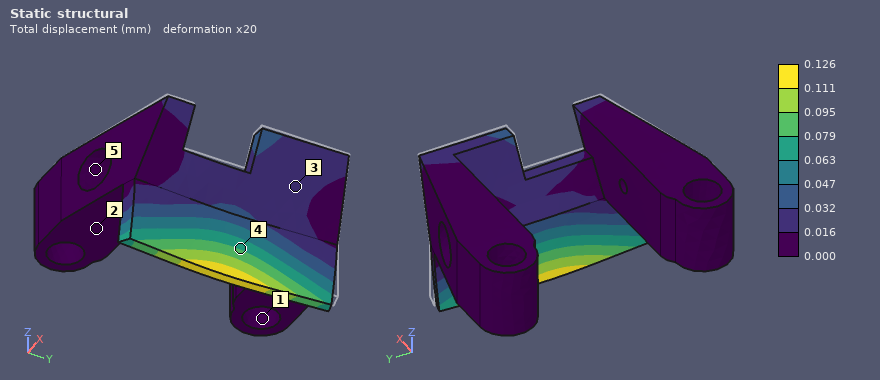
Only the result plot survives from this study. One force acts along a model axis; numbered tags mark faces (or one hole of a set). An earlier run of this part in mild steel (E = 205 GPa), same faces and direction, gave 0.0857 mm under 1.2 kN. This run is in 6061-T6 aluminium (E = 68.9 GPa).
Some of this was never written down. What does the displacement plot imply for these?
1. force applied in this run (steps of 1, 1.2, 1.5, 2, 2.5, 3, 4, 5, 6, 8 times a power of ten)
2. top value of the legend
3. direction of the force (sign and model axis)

600 N
0.126 mm
-X
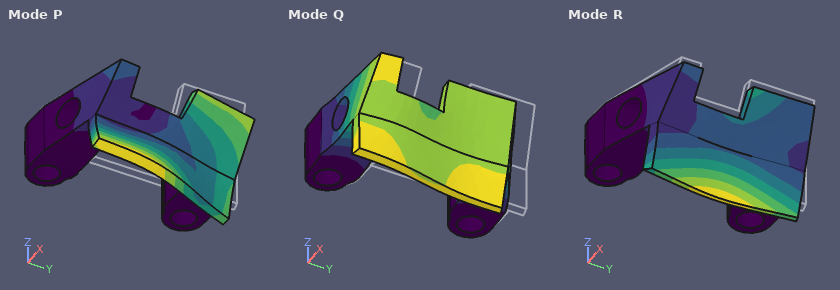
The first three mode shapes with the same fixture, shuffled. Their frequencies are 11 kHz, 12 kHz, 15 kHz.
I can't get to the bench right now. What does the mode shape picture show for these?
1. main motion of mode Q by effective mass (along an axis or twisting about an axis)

along Y
